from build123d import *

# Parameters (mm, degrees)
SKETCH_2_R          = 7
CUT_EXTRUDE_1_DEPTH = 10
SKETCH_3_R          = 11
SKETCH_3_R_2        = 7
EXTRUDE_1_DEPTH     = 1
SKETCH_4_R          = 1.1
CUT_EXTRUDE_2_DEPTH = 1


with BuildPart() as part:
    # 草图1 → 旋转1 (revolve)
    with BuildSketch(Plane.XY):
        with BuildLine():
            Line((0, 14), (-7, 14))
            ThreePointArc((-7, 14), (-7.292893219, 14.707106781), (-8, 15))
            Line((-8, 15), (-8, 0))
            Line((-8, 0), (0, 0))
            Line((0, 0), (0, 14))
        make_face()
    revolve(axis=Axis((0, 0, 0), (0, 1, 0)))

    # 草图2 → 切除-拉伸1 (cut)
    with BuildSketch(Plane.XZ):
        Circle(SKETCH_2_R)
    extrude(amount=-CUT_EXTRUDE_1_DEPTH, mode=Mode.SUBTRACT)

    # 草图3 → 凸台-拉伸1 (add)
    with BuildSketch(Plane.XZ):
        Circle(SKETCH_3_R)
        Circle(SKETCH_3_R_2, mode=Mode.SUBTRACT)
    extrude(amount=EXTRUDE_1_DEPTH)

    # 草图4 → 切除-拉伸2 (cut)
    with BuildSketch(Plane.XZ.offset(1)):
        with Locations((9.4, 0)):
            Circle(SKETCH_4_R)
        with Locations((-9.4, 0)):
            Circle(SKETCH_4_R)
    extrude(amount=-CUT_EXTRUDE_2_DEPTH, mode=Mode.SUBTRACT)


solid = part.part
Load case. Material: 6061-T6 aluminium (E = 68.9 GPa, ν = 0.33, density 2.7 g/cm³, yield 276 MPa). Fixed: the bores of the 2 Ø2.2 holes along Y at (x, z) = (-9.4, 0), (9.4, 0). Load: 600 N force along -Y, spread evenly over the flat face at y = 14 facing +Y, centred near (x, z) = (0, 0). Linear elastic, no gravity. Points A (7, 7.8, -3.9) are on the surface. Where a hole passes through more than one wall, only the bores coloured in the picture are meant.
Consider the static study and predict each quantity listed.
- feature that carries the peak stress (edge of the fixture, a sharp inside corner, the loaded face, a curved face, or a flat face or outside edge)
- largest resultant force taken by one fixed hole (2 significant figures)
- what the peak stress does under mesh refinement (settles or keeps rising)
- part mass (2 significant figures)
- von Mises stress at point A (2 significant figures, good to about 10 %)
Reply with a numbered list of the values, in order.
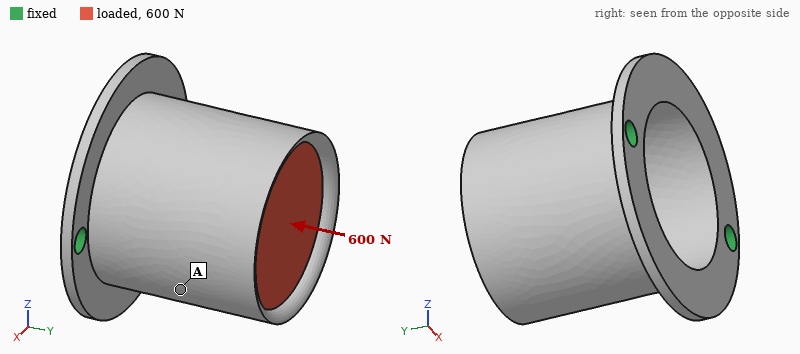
1. edge of the fixture
2. 310 N
3. keeps rising
4. 4.1 g
5. 19 MPa
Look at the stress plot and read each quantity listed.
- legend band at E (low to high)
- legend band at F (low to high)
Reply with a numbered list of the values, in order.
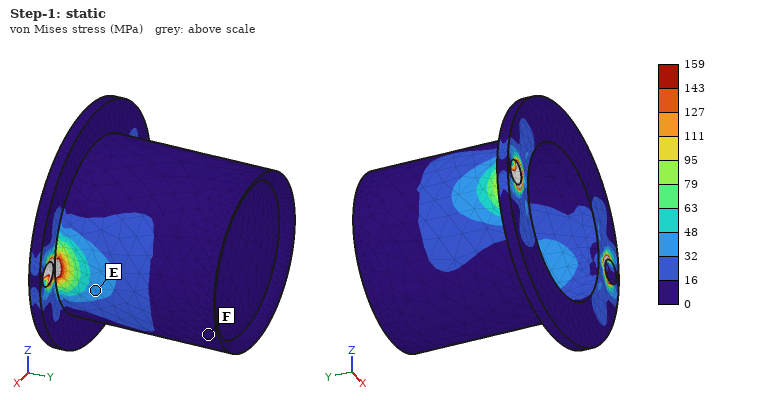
1. 32 to 48 MPa
2. 0 to 16 MPa
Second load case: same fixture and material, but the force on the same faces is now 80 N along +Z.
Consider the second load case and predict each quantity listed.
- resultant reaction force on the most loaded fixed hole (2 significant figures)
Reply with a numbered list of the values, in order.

1. 40 N
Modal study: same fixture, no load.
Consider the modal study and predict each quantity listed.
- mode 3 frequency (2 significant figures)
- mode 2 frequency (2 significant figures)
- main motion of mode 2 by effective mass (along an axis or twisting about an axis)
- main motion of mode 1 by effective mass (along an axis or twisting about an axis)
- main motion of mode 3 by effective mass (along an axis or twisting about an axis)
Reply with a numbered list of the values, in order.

1. 19 kHz
2. 12 kHz
3. along X
4. along Z
5. along Y
